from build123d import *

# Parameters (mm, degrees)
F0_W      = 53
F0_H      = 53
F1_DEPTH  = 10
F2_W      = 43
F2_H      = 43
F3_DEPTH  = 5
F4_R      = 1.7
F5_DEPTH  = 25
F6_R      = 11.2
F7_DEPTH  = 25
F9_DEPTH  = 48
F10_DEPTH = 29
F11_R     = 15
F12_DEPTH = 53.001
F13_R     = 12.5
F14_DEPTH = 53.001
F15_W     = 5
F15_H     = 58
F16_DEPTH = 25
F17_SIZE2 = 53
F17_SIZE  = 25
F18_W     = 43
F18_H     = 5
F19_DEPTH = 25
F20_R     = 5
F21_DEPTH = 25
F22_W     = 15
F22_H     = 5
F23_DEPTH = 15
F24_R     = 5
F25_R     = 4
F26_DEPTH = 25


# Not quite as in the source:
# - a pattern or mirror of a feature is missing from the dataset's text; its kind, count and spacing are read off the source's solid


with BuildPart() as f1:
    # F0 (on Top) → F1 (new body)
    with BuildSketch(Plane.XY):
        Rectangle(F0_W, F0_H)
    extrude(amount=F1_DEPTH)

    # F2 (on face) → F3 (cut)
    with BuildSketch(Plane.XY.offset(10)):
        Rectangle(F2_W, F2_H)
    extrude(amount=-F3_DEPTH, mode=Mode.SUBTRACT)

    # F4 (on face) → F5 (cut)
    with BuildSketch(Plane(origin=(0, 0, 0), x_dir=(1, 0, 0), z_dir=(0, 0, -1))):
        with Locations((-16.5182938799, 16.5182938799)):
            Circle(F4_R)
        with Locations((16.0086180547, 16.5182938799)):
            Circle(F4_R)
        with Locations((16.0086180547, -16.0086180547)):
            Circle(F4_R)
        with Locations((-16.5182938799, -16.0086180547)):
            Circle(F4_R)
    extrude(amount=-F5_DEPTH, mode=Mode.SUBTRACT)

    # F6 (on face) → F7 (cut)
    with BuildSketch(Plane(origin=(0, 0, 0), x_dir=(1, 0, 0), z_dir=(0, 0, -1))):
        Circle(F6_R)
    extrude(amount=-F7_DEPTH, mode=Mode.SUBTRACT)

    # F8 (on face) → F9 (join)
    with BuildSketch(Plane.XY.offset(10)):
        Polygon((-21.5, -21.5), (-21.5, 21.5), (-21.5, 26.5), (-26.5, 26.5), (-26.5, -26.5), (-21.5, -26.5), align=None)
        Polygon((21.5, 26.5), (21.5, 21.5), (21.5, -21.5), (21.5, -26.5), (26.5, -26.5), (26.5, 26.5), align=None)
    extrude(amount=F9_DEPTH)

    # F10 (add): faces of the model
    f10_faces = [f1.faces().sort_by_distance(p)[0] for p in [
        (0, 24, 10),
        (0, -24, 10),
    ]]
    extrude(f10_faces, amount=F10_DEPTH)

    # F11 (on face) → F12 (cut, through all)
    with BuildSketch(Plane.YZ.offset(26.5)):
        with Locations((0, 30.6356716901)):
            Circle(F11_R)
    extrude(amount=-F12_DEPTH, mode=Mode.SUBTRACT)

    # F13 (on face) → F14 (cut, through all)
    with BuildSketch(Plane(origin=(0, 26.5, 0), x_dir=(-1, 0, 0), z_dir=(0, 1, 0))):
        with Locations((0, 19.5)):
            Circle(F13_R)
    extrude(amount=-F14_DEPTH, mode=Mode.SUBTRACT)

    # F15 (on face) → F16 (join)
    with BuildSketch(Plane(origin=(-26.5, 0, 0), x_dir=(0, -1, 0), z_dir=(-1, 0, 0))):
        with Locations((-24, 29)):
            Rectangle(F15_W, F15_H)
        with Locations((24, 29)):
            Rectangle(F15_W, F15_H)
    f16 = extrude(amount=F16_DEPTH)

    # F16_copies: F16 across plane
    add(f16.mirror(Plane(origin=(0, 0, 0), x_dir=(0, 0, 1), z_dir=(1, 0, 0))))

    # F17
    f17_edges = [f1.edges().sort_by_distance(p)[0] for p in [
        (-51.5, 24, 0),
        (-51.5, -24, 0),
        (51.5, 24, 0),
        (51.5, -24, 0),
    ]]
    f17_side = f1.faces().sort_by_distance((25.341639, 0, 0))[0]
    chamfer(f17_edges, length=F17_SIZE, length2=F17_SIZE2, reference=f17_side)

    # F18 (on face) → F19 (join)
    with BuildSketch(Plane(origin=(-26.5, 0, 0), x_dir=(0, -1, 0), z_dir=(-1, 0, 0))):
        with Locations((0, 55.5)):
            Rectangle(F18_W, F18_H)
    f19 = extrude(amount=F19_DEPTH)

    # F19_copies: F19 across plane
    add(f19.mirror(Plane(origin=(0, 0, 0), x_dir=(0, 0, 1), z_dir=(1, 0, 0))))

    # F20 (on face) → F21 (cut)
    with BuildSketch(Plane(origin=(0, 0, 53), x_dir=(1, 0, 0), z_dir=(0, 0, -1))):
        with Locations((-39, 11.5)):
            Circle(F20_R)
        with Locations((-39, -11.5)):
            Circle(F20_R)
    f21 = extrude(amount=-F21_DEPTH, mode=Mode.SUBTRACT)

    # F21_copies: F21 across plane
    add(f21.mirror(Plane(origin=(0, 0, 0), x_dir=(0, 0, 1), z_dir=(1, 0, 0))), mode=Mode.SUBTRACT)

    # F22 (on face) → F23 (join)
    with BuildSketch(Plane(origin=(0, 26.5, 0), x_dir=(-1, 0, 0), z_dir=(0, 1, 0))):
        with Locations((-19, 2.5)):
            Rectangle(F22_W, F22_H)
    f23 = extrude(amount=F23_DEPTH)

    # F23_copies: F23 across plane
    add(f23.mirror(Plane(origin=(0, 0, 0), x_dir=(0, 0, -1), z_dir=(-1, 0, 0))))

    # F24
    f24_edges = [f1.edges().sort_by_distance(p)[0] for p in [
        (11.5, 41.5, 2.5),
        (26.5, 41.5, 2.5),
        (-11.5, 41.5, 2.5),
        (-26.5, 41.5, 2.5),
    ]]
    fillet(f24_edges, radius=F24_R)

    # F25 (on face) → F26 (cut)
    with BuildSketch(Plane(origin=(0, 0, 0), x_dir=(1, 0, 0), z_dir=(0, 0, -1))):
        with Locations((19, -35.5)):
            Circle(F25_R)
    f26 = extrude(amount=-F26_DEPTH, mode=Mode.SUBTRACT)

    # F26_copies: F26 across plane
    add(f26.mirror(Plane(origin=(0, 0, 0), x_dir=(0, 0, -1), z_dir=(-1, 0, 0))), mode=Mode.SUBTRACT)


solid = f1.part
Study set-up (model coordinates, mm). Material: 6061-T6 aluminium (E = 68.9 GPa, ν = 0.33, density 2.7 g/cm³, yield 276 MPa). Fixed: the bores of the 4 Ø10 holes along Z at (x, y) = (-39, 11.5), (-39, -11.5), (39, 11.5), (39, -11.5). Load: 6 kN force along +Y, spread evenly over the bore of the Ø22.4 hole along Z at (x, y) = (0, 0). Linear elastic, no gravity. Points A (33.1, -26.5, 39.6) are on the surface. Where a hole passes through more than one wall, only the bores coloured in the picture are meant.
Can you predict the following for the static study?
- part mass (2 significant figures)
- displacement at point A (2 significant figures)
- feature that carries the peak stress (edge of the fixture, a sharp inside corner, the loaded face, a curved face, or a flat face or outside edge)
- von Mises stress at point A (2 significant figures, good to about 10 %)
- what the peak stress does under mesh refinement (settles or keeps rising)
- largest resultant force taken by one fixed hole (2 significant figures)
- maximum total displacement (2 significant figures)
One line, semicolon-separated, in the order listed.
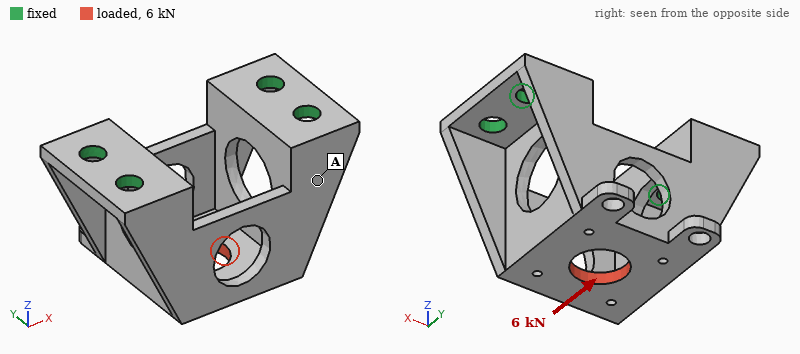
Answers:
190 g; 0.098 mm; edge of the fixture; 40 MPa; keeps rising; 5.2 kN; 0.26 mm
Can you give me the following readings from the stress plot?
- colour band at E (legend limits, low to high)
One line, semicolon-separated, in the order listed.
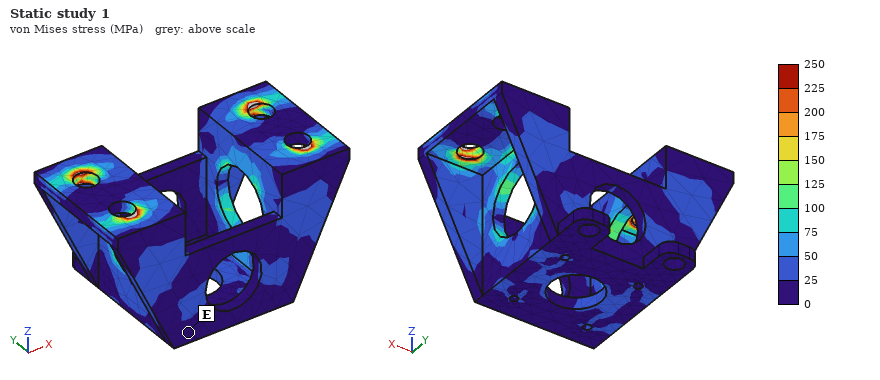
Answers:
0 to 25 MPa
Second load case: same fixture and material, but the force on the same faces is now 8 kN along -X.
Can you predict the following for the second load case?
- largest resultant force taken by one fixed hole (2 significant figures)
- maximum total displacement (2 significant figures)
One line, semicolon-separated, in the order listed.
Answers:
3.3 kN; 0.15 mm
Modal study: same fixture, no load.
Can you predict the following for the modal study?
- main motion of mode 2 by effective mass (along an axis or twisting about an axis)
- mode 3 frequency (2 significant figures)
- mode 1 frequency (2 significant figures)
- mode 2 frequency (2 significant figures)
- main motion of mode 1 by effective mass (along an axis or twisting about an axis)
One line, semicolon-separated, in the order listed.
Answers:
along X; 4600 Hz; 2800 Hz; 4100 Hz; along Y
